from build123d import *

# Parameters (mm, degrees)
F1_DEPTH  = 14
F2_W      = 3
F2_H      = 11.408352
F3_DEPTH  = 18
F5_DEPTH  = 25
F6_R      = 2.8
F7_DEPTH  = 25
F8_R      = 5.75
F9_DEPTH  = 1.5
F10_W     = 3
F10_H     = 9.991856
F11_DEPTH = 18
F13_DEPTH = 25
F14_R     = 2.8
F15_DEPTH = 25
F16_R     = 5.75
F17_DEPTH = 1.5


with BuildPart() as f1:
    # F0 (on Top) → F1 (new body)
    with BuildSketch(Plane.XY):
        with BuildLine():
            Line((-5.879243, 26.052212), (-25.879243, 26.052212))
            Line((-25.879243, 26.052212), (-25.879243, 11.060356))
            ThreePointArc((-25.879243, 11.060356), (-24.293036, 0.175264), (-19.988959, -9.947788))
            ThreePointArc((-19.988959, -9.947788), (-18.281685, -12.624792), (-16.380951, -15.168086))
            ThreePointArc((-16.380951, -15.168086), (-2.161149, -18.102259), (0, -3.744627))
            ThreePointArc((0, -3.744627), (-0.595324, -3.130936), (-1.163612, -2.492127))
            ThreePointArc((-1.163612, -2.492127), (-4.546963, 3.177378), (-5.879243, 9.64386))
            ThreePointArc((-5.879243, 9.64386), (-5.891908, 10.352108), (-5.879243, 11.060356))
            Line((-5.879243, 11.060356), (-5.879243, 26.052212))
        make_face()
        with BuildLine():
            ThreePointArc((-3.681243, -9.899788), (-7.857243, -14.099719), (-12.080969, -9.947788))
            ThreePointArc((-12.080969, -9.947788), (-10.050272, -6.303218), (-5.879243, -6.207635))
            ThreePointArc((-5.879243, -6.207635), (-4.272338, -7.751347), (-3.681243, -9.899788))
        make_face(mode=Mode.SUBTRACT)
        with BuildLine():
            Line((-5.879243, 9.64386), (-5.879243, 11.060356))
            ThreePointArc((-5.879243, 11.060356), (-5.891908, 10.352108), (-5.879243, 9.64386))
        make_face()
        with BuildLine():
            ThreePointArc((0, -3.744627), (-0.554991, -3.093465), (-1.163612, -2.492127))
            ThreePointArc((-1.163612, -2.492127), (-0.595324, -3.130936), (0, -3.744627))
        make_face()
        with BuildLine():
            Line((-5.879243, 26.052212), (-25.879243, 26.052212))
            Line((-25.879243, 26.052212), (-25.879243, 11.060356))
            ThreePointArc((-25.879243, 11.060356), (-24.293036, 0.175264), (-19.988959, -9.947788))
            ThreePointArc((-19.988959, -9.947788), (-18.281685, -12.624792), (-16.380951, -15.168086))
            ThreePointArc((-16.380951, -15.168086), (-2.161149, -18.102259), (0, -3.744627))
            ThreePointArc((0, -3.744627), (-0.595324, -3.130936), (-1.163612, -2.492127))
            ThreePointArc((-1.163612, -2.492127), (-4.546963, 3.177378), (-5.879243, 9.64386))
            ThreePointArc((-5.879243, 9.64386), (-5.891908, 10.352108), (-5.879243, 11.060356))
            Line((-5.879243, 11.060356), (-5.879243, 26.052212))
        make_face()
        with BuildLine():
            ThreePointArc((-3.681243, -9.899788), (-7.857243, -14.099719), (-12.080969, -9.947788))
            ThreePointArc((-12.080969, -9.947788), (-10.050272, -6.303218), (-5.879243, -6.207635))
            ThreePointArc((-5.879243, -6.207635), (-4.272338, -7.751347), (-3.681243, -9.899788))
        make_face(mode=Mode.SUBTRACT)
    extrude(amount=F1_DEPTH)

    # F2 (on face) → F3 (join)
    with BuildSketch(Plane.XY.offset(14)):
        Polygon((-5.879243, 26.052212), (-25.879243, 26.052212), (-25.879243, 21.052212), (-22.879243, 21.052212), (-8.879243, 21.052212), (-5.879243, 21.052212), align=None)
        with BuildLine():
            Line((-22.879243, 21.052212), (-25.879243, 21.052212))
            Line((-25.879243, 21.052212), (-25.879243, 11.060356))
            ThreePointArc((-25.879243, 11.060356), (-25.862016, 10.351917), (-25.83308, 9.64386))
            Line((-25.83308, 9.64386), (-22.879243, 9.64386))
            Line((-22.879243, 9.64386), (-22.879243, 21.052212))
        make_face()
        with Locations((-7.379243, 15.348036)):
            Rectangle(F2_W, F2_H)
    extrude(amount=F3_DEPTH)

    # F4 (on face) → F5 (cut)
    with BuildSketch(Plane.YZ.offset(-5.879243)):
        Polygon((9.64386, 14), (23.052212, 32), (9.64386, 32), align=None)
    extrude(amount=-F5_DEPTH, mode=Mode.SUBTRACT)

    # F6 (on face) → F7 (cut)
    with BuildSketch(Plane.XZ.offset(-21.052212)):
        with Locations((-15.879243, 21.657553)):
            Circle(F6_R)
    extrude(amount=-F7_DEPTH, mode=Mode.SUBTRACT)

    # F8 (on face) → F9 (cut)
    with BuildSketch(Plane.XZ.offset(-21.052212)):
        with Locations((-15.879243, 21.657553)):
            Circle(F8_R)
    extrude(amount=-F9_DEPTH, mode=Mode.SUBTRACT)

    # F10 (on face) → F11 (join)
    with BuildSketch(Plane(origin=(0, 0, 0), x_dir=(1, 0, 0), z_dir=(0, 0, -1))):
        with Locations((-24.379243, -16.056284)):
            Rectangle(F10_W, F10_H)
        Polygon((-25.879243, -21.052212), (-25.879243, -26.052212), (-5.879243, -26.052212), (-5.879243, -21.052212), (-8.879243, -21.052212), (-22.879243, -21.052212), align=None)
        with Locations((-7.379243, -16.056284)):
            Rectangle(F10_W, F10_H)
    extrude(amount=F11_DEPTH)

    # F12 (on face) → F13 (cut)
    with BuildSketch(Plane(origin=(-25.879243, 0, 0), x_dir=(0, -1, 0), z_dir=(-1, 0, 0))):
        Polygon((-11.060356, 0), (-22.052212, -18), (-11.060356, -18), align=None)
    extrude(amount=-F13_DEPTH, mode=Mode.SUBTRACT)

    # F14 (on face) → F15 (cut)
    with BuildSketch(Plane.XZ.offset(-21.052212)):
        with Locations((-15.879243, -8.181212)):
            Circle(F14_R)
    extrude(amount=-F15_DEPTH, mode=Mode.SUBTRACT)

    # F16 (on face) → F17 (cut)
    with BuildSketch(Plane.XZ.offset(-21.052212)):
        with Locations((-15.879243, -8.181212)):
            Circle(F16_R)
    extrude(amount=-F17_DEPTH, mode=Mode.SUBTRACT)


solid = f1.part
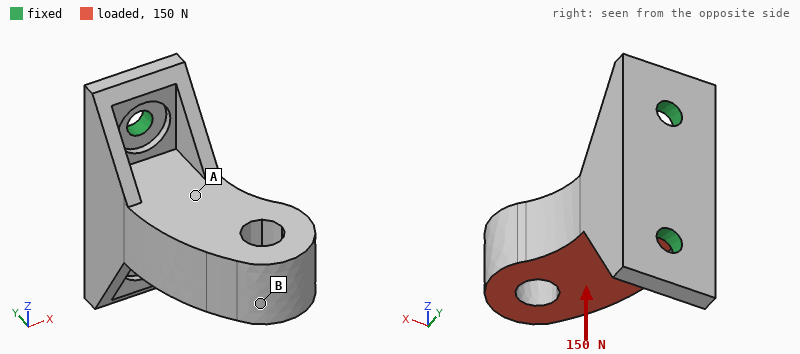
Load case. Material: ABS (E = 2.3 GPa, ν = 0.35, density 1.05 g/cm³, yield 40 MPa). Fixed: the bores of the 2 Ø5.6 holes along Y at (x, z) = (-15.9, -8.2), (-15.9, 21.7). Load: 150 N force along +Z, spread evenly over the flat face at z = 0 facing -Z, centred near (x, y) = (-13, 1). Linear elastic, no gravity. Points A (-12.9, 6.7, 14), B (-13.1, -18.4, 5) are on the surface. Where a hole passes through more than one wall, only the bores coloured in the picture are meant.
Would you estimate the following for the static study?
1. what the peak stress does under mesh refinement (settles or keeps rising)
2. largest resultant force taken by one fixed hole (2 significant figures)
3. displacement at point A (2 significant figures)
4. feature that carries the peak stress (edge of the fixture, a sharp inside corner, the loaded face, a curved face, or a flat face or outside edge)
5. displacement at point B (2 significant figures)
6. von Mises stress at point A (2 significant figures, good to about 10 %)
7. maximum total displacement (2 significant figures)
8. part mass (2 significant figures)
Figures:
keeps rising
150 N
0.060 mm
edge of the fixture
0.18 mm
1.8 MPa
0.19 mm
17 g
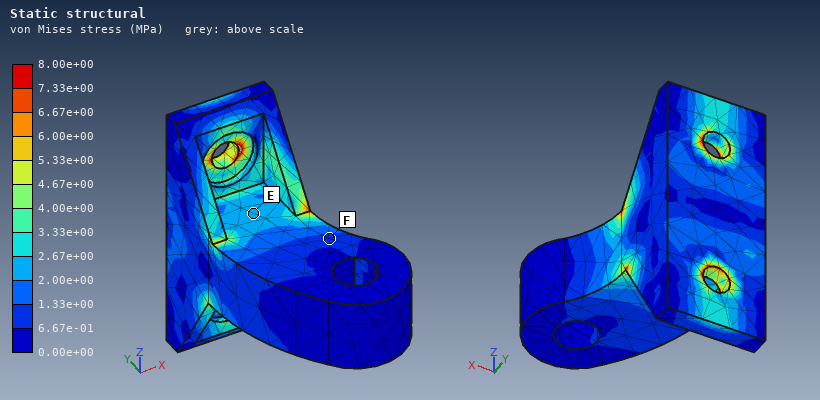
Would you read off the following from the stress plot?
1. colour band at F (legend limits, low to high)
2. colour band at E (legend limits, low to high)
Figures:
6.67e-01 to 1.33e+00 MPa
2.00e+00 to 2.67e+00 MPa
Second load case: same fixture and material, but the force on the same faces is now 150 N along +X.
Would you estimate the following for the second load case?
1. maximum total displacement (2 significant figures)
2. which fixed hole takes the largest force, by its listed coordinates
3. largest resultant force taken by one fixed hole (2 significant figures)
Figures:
0.79 mm
(-15.9, -8.2)
110 N
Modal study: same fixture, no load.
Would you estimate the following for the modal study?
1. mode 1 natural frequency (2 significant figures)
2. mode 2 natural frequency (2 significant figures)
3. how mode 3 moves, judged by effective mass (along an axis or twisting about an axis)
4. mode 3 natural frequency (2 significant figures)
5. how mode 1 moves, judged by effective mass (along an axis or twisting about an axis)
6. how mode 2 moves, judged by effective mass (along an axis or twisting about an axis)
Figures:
820 Hz
1700 Hz
along Y
3700 Hz
along X
along Z
